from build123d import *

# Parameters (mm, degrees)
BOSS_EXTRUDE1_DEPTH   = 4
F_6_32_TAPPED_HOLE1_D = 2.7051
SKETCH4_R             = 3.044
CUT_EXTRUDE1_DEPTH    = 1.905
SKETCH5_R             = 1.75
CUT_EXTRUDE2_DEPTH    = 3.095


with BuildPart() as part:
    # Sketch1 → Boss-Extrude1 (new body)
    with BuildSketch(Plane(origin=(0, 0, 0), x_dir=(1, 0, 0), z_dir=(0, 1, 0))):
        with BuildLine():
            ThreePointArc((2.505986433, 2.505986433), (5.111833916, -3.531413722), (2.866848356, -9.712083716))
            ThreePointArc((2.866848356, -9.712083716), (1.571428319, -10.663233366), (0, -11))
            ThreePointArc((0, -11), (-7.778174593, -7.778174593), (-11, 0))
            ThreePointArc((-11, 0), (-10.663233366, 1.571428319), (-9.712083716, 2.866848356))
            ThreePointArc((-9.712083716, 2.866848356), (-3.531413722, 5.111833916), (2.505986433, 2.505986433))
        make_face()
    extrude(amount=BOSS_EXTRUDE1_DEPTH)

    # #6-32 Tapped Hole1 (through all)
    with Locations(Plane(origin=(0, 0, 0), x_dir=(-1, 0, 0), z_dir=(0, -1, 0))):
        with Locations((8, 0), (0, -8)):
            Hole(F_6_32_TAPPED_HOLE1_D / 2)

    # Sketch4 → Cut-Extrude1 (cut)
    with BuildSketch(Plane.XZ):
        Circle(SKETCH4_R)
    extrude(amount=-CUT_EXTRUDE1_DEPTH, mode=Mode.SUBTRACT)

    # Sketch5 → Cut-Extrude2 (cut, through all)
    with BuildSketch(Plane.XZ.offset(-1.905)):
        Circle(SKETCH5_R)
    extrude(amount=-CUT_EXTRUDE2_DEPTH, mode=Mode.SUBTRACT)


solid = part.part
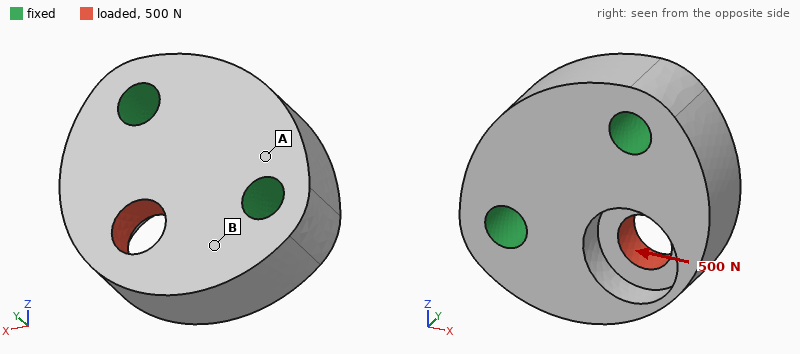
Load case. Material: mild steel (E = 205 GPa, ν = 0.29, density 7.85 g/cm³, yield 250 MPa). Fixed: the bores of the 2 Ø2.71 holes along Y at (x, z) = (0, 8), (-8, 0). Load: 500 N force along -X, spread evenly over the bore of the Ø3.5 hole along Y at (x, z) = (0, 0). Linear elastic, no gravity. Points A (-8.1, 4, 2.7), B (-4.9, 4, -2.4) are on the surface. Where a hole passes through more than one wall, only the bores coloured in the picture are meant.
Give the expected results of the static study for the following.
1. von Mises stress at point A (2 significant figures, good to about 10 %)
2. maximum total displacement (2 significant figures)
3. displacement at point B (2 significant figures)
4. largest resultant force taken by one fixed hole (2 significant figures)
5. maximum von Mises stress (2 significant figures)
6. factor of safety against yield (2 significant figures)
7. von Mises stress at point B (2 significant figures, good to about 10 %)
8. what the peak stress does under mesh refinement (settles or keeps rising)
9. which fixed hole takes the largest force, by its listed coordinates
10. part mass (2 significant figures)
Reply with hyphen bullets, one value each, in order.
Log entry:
- 8.5 MPa
- 1.7 µm
- 0.48 µm
- 380 N
- 65 MPa
- 3.9
- 24 MPa
- settles
- (-8, 0)
- 5.3 g
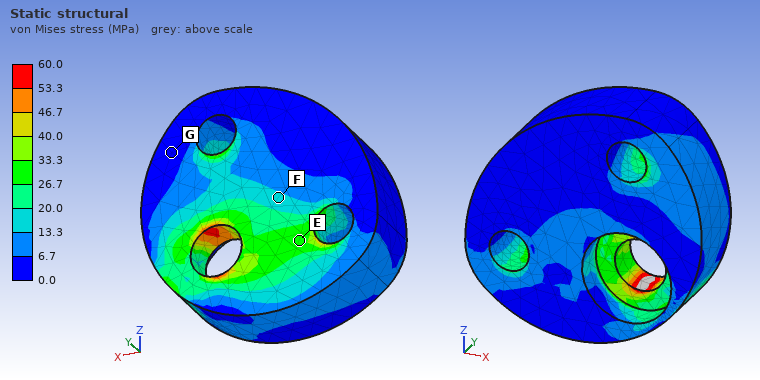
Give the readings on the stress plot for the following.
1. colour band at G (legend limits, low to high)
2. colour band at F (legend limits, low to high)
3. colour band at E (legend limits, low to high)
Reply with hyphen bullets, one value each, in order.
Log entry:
- 0.0 to 6.7 MPa
- 13.3 to 20.0 MPa
- 26.7 to 33.3 MPa
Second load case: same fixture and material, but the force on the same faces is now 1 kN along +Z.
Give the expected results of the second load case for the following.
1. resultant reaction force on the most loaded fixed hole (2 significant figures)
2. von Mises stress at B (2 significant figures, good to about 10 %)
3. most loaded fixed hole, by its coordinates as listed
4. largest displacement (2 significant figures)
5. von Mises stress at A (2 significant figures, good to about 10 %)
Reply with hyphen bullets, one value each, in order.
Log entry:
- 770 N
- 18 MPa
- (0, 8)
- 3.3 µm
- 14 MPa
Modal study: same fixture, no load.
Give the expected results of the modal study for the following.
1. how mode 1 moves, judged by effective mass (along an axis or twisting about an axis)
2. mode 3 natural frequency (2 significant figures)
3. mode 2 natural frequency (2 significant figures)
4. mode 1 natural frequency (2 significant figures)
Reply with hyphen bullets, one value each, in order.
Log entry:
- along Y
- 88 kHz
- 76 kHz
- 47 kHz
